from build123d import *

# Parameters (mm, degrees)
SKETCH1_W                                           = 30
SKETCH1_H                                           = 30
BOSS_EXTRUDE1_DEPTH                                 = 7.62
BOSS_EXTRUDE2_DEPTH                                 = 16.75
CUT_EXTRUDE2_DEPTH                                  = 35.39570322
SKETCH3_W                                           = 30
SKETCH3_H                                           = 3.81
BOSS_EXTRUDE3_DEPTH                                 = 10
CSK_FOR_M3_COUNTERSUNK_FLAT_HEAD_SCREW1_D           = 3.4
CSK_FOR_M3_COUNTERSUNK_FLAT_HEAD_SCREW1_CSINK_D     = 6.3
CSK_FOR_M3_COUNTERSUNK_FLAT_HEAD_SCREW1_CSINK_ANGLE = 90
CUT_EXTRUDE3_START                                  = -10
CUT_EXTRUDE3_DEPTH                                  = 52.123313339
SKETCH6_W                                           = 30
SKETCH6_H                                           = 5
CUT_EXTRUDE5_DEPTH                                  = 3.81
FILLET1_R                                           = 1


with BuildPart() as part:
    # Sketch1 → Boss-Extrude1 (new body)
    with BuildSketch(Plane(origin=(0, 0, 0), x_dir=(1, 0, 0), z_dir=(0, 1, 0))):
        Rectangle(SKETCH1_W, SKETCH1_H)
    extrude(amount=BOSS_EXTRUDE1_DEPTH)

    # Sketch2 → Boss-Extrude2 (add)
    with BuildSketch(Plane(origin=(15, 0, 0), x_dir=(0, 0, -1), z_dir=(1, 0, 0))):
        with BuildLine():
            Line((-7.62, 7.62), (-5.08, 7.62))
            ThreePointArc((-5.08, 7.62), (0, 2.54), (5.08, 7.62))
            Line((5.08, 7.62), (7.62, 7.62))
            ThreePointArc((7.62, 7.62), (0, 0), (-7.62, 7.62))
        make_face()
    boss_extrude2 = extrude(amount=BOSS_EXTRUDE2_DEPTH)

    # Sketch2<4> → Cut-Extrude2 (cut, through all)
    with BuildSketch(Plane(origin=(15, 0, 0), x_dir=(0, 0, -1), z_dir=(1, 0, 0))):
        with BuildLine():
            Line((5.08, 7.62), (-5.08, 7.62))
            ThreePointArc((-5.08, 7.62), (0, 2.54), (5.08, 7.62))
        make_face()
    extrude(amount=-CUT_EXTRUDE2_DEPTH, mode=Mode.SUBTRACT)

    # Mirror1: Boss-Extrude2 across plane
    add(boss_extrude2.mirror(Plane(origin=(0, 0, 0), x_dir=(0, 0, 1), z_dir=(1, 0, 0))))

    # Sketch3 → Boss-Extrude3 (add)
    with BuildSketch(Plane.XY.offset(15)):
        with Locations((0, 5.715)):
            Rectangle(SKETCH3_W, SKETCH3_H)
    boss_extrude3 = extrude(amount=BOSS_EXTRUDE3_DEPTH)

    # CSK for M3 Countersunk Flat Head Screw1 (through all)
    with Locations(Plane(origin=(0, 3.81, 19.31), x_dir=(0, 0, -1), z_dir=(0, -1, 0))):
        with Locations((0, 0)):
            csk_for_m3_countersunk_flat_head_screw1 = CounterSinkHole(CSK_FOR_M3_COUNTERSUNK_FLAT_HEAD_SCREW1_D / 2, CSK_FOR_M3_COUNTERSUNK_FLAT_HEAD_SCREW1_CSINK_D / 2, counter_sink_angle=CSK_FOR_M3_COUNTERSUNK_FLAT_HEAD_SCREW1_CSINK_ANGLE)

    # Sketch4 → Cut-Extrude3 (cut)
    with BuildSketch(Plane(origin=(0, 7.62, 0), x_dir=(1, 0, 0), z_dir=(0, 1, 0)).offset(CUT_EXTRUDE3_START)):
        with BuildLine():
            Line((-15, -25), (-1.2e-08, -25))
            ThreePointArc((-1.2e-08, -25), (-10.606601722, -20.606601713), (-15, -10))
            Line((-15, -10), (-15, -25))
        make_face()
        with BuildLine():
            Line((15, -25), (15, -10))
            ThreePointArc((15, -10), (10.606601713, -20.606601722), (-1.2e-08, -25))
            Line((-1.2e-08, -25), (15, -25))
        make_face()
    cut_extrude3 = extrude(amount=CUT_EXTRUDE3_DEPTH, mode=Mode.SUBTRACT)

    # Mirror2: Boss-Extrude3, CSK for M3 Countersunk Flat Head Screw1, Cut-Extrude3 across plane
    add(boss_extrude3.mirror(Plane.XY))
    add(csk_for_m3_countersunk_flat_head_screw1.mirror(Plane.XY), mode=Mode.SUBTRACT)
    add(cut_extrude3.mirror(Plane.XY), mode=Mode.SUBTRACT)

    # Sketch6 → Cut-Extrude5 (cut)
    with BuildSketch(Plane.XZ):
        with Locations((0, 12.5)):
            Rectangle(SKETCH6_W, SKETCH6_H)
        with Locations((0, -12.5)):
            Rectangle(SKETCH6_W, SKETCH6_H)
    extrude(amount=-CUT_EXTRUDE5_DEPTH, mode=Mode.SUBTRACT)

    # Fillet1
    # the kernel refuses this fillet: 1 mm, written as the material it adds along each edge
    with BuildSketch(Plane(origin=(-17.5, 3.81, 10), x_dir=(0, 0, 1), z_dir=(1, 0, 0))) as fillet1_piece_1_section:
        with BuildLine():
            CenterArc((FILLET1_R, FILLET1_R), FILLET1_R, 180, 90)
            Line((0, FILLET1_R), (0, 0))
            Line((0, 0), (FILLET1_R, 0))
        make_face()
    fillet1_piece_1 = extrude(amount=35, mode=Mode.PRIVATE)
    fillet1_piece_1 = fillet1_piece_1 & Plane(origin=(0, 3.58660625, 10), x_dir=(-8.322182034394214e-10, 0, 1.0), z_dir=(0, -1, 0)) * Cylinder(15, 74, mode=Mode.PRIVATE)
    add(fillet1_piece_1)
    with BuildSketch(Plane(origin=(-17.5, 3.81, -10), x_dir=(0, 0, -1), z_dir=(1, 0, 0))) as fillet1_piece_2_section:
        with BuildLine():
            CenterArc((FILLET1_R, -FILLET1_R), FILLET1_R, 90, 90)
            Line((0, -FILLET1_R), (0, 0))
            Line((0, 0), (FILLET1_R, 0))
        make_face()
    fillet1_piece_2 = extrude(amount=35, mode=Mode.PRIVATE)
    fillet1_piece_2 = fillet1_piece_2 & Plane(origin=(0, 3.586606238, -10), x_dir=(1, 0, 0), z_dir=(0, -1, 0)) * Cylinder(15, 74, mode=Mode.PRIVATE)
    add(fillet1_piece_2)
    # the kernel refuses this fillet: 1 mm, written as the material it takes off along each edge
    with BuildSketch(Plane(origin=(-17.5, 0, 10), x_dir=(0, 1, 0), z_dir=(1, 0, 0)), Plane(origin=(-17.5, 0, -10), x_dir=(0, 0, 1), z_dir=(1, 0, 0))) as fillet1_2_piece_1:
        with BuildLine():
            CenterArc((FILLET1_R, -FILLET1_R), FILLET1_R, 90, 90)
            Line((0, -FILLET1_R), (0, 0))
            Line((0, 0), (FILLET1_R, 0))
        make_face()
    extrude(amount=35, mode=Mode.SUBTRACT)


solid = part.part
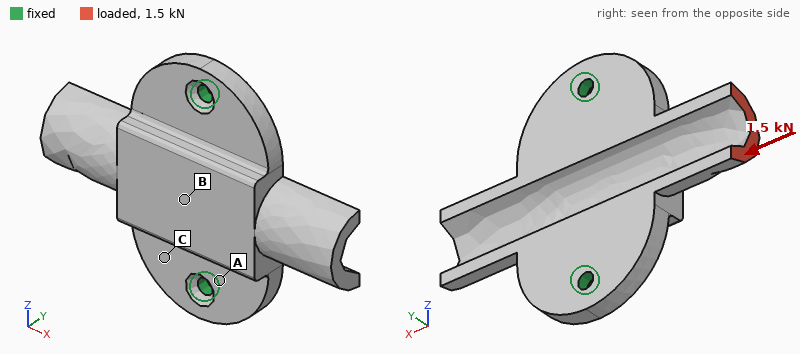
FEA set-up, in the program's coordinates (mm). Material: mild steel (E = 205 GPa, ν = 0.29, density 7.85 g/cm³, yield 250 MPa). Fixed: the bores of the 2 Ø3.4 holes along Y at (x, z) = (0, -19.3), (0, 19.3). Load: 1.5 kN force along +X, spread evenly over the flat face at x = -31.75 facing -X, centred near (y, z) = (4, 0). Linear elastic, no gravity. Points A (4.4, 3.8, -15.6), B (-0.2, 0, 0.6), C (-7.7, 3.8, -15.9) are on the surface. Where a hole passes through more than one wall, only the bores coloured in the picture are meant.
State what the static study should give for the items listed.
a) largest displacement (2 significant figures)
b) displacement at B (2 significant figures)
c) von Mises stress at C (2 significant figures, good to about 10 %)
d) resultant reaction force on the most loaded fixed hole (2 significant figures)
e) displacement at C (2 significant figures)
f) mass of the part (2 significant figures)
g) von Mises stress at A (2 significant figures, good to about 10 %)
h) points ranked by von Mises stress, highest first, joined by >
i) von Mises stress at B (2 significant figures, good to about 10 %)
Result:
35 µm
9.2 µm
24 MPa
750 N
5.5 µm
60 g
31 MPa
A > C > B
9.6 MPa
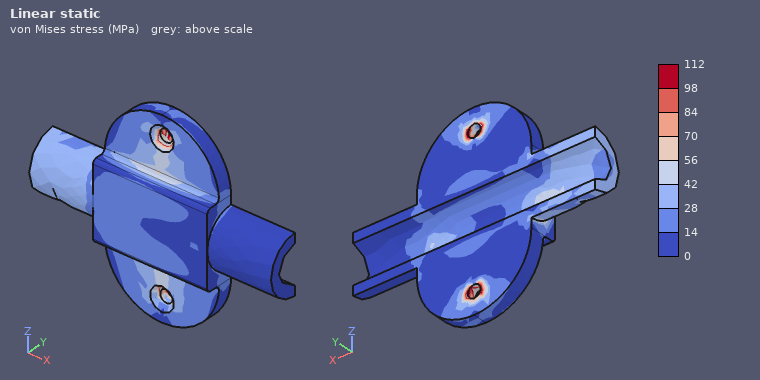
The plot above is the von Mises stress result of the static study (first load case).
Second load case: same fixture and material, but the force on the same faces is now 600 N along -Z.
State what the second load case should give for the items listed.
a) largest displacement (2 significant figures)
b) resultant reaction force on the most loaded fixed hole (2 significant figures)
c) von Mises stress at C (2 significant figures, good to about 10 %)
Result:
43 µm
580 N
13 MPa
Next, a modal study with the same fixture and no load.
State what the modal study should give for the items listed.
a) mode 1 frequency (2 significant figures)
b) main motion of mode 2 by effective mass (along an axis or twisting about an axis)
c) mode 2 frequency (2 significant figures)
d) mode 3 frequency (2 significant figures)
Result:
3200 Hz
along Y
6900 Hz
12 kHz
